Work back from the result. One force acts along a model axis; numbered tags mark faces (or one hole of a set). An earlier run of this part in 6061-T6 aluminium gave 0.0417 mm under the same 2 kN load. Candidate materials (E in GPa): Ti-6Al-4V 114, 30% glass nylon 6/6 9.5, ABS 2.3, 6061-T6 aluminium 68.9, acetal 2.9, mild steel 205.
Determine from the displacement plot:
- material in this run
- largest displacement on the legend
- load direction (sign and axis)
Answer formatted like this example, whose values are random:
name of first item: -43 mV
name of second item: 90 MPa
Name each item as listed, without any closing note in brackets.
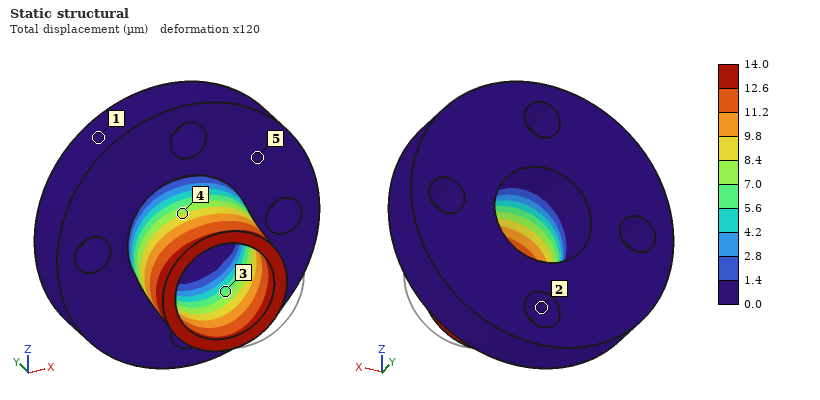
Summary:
material in this run: mild steel
largest displacement on the legend: 14.0 µm
load direction: -X
